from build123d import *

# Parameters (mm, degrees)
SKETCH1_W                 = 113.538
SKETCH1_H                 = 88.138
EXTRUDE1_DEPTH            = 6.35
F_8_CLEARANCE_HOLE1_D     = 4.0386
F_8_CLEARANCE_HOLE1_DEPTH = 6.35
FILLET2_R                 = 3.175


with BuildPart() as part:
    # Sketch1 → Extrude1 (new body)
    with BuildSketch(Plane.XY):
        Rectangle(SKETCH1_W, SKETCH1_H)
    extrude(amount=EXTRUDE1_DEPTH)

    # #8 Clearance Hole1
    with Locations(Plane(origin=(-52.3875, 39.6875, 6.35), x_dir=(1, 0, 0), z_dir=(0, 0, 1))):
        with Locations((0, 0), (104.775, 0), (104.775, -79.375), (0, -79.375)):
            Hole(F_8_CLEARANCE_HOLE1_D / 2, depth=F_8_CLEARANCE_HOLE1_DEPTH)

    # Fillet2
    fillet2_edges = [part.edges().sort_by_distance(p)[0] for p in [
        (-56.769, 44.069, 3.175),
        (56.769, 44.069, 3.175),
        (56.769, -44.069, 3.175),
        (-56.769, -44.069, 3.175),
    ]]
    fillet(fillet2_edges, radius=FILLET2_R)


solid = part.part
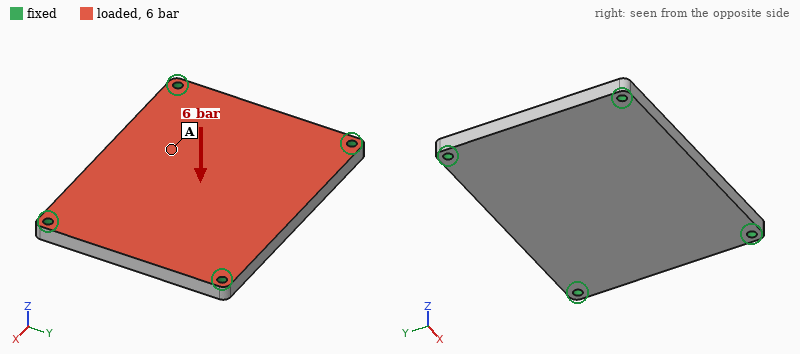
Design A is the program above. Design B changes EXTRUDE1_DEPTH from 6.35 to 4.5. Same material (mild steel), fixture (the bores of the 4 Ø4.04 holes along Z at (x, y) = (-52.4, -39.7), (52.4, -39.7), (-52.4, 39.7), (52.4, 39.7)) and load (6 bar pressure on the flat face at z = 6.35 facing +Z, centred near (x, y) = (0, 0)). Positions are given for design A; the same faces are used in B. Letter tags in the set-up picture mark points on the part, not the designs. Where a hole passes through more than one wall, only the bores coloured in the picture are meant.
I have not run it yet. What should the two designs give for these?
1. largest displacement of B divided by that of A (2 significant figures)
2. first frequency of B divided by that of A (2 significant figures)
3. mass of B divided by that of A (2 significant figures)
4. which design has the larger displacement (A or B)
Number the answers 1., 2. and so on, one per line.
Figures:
1. 2.6
2. 0.73
3. 0.71
4. B
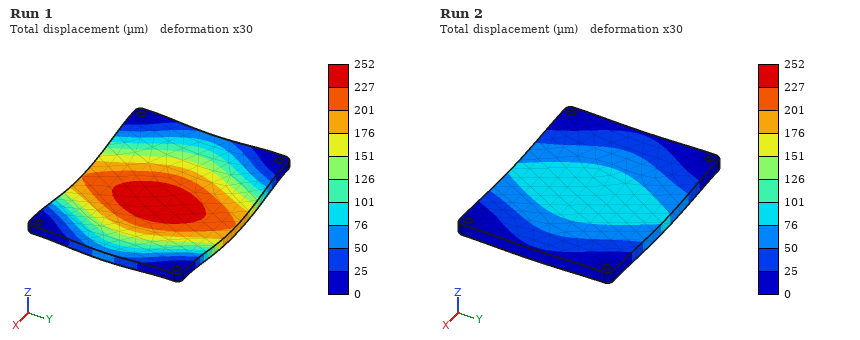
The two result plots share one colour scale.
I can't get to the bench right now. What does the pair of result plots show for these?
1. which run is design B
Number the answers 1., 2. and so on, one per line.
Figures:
1. Run 1
